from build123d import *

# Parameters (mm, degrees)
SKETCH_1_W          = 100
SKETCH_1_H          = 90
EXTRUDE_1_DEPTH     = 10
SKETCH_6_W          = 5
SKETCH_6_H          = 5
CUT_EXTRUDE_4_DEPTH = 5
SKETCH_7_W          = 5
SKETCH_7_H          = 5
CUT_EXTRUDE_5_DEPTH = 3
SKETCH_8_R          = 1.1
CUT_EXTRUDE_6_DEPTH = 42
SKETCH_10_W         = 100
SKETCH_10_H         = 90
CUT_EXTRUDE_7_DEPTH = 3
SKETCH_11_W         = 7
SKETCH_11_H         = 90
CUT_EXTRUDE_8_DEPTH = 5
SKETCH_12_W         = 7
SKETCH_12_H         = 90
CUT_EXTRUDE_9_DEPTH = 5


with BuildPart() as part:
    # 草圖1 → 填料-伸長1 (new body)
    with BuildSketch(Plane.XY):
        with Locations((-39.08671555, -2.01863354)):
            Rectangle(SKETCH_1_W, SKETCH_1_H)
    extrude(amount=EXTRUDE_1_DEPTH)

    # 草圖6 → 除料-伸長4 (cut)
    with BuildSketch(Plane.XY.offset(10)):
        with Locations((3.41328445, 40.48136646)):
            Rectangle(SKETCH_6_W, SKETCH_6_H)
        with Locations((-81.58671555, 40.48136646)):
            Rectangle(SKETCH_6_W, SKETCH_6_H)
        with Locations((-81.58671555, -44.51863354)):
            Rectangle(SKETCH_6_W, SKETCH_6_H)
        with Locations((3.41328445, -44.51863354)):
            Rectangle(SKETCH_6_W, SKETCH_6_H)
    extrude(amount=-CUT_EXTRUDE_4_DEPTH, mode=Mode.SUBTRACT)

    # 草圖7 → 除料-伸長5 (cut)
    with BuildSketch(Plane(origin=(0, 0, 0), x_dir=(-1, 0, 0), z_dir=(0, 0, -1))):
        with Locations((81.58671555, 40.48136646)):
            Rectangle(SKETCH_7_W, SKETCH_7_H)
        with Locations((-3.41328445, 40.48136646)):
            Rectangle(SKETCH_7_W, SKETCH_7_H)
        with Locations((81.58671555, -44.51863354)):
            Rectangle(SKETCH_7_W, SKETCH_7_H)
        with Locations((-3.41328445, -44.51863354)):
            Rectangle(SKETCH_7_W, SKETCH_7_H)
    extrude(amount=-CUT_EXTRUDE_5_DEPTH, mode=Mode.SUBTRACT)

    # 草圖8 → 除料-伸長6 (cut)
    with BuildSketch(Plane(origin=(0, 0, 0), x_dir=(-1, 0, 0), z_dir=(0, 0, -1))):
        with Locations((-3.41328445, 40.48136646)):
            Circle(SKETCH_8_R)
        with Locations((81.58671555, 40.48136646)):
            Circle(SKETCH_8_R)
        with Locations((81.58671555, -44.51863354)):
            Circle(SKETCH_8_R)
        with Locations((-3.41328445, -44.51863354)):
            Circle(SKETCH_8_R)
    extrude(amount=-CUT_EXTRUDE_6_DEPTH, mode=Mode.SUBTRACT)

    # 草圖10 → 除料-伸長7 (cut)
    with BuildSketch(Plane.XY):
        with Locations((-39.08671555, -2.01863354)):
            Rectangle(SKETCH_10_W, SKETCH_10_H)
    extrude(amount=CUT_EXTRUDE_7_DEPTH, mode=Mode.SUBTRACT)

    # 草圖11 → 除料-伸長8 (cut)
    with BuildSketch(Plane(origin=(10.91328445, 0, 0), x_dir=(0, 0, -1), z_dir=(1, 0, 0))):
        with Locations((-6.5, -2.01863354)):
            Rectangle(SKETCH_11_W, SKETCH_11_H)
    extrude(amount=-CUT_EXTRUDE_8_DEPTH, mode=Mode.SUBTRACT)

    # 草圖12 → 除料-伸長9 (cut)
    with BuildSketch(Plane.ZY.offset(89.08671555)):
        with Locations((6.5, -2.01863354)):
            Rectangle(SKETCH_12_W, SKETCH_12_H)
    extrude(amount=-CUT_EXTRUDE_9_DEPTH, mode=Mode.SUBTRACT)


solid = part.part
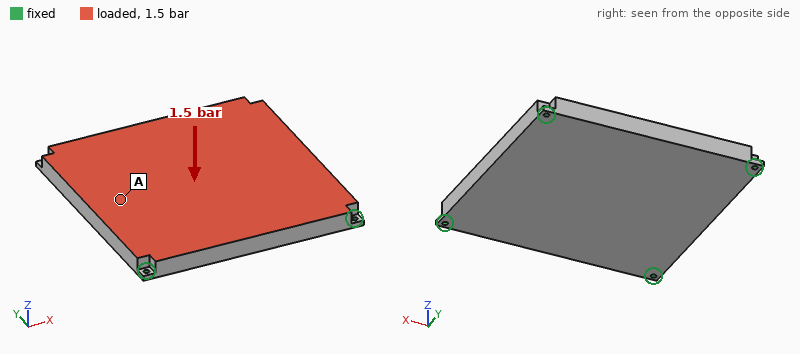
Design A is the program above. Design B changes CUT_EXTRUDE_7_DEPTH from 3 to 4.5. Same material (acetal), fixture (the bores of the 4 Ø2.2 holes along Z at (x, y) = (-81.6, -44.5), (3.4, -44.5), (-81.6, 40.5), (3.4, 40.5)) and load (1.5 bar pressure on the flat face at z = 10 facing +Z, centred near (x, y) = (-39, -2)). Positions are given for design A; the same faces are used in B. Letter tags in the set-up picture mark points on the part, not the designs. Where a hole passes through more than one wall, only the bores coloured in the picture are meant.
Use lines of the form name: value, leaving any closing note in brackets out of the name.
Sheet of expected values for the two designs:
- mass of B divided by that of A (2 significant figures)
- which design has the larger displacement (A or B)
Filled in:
mass of B divided by that of A: 0.78
which design has the larger displacement: B
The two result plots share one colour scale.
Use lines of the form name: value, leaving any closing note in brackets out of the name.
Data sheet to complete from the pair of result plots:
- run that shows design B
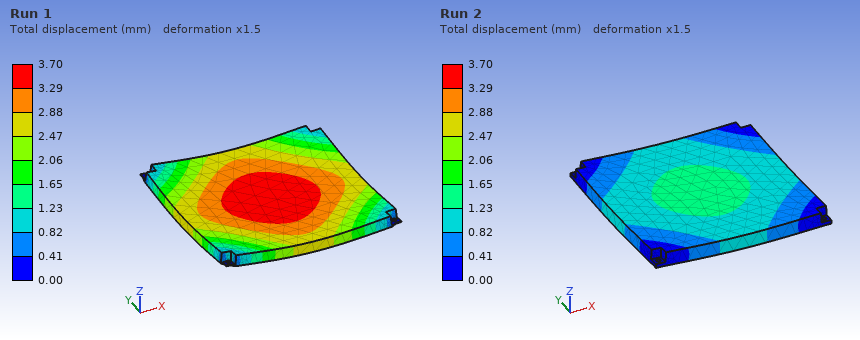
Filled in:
run that shows design B: Run 1
